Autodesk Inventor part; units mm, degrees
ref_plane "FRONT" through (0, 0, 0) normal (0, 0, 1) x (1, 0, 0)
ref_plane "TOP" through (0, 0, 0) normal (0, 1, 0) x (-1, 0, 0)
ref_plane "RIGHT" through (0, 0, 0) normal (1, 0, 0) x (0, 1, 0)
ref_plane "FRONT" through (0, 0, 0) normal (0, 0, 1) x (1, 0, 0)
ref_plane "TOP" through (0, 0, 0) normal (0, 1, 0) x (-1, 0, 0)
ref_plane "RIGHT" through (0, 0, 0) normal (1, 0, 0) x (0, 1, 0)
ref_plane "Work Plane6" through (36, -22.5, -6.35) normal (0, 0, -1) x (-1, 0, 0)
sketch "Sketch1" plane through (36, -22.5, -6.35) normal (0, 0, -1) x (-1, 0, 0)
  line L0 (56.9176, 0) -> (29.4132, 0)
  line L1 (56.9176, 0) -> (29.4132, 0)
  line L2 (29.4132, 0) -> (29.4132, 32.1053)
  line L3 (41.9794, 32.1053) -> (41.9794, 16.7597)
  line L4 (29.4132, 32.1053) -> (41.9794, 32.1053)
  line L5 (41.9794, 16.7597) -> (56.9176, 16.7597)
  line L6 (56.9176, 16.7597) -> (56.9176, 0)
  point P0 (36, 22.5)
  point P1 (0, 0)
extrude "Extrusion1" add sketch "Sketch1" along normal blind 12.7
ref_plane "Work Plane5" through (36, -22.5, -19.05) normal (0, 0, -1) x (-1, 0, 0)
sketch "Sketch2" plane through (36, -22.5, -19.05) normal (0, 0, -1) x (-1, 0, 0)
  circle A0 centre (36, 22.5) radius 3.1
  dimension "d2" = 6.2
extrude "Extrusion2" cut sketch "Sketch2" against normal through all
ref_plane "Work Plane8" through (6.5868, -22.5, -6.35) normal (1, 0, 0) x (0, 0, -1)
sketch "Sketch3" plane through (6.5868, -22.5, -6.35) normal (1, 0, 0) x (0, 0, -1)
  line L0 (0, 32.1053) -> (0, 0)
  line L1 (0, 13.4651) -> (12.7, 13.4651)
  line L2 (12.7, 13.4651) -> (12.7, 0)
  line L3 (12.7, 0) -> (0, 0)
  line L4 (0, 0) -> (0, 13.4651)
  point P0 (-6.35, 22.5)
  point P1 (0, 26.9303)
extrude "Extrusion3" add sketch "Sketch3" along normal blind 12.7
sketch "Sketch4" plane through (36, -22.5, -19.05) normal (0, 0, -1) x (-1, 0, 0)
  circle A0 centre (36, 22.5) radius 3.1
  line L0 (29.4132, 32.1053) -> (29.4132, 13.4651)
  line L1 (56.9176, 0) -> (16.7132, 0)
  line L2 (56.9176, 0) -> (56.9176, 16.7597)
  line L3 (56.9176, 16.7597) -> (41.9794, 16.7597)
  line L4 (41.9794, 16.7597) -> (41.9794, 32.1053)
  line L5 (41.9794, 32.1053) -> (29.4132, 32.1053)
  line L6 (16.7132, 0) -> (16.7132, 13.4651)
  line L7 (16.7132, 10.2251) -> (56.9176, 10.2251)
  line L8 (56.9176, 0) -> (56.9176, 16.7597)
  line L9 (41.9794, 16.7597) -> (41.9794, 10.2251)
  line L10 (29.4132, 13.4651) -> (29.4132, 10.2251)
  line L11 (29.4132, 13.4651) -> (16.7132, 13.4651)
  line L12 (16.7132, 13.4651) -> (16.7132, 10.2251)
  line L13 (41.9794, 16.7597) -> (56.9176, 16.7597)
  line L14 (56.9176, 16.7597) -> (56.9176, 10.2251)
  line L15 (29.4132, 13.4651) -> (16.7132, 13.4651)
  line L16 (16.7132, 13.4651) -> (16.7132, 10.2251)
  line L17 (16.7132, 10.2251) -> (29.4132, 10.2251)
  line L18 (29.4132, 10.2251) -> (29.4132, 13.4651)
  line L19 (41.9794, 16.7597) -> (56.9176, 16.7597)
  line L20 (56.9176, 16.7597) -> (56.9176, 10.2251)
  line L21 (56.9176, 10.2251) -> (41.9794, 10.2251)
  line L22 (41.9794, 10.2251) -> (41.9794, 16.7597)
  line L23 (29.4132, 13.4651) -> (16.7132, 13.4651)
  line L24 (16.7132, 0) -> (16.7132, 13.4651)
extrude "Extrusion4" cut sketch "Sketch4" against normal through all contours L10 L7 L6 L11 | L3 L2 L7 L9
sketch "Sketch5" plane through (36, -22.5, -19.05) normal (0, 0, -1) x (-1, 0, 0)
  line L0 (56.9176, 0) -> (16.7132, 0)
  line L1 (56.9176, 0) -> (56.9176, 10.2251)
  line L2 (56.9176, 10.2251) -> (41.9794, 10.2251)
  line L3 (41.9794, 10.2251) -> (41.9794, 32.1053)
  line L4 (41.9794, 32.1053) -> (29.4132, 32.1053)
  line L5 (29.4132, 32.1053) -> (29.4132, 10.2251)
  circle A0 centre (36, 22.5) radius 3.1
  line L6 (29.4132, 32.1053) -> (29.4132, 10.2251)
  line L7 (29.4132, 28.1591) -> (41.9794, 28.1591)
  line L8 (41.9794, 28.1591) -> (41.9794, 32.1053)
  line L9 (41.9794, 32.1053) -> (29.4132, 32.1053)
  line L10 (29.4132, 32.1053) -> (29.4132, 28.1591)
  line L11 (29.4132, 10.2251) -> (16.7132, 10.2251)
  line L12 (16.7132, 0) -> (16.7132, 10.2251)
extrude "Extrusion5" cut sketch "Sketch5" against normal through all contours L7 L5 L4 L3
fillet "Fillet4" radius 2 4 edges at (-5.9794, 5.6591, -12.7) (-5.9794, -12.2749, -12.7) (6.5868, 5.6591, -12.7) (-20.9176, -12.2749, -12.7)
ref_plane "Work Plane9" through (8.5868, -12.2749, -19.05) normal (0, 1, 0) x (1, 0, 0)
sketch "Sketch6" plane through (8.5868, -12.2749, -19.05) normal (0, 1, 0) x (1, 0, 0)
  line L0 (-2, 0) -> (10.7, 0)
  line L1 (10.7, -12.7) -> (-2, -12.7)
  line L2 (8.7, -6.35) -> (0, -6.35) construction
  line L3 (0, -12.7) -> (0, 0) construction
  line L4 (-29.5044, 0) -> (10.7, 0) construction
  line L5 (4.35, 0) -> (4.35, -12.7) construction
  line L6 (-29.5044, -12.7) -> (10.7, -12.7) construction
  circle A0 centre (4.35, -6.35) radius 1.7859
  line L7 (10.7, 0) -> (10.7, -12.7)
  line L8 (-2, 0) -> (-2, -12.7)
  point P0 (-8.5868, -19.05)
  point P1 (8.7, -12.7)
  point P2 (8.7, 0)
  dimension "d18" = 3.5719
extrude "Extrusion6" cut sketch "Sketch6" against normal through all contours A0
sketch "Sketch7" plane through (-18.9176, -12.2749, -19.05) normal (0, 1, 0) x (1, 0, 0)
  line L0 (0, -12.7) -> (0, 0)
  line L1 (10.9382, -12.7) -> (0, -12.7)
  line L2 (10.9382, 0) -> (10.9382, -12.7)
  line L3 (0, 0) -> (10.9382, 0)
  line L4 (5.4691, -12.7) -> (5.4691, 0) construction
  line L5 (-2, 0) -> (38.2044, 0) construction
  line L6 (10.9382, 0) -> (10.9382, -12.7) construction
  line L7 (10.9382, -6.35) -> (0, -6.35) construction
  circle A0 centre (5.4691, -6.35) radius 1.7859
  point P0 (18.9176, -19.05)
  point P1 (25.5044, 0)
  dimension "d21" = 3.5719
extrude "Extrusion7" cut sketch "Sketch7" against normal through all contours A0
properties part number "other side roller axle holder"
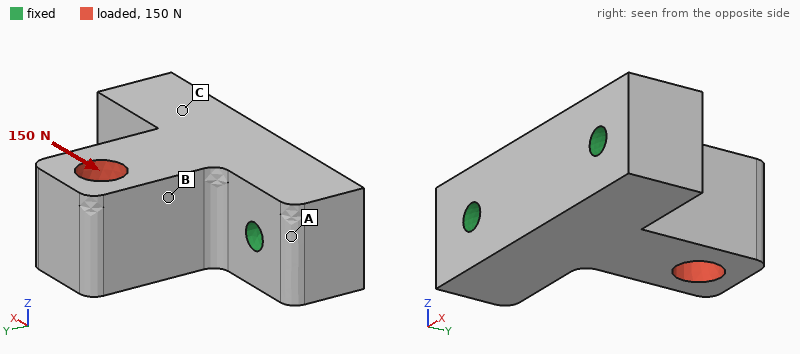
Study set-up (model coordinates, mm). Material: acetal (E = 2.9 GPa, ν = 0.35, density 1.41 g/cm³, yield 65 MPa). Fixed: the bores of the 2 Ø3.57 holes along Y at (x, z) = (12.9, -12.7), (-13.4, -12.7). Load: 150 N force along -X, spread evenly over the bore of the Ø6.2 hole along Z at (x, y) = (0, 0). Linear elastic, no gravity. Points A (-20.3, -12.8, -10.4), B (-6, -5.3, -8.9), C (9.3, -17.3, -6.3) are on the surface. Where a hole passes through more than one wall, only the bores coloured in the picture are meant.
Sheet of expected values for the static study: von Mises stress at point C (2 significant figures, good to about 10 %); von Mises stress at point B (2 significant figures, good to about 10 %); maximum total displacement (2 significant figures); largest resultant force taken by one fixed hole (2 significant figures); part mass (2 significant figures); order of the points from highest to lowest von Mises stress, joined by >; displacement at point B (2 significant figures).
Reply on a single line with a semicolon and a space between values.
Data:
1.9 MPa; 3.4 MPa; 83 µm; 140 N; 11 g; B > C > A; 34 µm
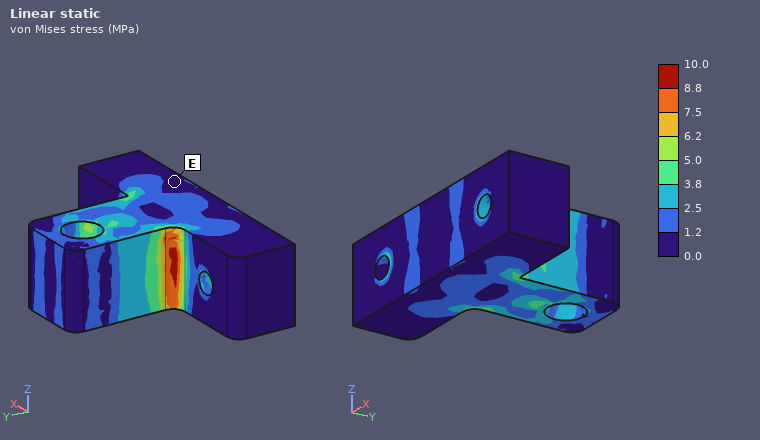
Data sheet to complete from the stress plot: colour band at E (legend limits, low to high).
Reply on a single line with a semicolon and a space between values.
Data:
0.0 to 1.2 MPa
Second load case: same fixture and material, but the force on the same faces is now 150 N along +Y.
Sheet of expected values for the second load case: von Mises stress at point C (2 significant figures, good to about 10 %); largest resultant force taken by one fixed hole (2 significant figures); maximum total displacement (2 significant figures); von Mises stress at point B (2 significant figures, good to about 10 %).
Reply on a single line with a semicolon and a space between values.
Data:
1.1 MPa; 79 N; 16 µm; 1.4 MPa
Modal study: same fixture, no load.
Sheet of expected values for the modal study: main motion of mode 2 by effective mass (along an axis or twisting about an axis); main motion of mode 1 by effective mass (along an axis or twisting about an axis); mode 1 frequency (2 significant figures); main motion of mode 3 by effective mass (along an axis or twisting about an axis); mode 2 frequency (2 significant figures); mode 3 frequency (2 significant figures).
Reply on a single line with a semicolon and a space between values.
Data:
along X; along Z; 3400 Hz; along Y; 5300 Hz; 8800 Hz
